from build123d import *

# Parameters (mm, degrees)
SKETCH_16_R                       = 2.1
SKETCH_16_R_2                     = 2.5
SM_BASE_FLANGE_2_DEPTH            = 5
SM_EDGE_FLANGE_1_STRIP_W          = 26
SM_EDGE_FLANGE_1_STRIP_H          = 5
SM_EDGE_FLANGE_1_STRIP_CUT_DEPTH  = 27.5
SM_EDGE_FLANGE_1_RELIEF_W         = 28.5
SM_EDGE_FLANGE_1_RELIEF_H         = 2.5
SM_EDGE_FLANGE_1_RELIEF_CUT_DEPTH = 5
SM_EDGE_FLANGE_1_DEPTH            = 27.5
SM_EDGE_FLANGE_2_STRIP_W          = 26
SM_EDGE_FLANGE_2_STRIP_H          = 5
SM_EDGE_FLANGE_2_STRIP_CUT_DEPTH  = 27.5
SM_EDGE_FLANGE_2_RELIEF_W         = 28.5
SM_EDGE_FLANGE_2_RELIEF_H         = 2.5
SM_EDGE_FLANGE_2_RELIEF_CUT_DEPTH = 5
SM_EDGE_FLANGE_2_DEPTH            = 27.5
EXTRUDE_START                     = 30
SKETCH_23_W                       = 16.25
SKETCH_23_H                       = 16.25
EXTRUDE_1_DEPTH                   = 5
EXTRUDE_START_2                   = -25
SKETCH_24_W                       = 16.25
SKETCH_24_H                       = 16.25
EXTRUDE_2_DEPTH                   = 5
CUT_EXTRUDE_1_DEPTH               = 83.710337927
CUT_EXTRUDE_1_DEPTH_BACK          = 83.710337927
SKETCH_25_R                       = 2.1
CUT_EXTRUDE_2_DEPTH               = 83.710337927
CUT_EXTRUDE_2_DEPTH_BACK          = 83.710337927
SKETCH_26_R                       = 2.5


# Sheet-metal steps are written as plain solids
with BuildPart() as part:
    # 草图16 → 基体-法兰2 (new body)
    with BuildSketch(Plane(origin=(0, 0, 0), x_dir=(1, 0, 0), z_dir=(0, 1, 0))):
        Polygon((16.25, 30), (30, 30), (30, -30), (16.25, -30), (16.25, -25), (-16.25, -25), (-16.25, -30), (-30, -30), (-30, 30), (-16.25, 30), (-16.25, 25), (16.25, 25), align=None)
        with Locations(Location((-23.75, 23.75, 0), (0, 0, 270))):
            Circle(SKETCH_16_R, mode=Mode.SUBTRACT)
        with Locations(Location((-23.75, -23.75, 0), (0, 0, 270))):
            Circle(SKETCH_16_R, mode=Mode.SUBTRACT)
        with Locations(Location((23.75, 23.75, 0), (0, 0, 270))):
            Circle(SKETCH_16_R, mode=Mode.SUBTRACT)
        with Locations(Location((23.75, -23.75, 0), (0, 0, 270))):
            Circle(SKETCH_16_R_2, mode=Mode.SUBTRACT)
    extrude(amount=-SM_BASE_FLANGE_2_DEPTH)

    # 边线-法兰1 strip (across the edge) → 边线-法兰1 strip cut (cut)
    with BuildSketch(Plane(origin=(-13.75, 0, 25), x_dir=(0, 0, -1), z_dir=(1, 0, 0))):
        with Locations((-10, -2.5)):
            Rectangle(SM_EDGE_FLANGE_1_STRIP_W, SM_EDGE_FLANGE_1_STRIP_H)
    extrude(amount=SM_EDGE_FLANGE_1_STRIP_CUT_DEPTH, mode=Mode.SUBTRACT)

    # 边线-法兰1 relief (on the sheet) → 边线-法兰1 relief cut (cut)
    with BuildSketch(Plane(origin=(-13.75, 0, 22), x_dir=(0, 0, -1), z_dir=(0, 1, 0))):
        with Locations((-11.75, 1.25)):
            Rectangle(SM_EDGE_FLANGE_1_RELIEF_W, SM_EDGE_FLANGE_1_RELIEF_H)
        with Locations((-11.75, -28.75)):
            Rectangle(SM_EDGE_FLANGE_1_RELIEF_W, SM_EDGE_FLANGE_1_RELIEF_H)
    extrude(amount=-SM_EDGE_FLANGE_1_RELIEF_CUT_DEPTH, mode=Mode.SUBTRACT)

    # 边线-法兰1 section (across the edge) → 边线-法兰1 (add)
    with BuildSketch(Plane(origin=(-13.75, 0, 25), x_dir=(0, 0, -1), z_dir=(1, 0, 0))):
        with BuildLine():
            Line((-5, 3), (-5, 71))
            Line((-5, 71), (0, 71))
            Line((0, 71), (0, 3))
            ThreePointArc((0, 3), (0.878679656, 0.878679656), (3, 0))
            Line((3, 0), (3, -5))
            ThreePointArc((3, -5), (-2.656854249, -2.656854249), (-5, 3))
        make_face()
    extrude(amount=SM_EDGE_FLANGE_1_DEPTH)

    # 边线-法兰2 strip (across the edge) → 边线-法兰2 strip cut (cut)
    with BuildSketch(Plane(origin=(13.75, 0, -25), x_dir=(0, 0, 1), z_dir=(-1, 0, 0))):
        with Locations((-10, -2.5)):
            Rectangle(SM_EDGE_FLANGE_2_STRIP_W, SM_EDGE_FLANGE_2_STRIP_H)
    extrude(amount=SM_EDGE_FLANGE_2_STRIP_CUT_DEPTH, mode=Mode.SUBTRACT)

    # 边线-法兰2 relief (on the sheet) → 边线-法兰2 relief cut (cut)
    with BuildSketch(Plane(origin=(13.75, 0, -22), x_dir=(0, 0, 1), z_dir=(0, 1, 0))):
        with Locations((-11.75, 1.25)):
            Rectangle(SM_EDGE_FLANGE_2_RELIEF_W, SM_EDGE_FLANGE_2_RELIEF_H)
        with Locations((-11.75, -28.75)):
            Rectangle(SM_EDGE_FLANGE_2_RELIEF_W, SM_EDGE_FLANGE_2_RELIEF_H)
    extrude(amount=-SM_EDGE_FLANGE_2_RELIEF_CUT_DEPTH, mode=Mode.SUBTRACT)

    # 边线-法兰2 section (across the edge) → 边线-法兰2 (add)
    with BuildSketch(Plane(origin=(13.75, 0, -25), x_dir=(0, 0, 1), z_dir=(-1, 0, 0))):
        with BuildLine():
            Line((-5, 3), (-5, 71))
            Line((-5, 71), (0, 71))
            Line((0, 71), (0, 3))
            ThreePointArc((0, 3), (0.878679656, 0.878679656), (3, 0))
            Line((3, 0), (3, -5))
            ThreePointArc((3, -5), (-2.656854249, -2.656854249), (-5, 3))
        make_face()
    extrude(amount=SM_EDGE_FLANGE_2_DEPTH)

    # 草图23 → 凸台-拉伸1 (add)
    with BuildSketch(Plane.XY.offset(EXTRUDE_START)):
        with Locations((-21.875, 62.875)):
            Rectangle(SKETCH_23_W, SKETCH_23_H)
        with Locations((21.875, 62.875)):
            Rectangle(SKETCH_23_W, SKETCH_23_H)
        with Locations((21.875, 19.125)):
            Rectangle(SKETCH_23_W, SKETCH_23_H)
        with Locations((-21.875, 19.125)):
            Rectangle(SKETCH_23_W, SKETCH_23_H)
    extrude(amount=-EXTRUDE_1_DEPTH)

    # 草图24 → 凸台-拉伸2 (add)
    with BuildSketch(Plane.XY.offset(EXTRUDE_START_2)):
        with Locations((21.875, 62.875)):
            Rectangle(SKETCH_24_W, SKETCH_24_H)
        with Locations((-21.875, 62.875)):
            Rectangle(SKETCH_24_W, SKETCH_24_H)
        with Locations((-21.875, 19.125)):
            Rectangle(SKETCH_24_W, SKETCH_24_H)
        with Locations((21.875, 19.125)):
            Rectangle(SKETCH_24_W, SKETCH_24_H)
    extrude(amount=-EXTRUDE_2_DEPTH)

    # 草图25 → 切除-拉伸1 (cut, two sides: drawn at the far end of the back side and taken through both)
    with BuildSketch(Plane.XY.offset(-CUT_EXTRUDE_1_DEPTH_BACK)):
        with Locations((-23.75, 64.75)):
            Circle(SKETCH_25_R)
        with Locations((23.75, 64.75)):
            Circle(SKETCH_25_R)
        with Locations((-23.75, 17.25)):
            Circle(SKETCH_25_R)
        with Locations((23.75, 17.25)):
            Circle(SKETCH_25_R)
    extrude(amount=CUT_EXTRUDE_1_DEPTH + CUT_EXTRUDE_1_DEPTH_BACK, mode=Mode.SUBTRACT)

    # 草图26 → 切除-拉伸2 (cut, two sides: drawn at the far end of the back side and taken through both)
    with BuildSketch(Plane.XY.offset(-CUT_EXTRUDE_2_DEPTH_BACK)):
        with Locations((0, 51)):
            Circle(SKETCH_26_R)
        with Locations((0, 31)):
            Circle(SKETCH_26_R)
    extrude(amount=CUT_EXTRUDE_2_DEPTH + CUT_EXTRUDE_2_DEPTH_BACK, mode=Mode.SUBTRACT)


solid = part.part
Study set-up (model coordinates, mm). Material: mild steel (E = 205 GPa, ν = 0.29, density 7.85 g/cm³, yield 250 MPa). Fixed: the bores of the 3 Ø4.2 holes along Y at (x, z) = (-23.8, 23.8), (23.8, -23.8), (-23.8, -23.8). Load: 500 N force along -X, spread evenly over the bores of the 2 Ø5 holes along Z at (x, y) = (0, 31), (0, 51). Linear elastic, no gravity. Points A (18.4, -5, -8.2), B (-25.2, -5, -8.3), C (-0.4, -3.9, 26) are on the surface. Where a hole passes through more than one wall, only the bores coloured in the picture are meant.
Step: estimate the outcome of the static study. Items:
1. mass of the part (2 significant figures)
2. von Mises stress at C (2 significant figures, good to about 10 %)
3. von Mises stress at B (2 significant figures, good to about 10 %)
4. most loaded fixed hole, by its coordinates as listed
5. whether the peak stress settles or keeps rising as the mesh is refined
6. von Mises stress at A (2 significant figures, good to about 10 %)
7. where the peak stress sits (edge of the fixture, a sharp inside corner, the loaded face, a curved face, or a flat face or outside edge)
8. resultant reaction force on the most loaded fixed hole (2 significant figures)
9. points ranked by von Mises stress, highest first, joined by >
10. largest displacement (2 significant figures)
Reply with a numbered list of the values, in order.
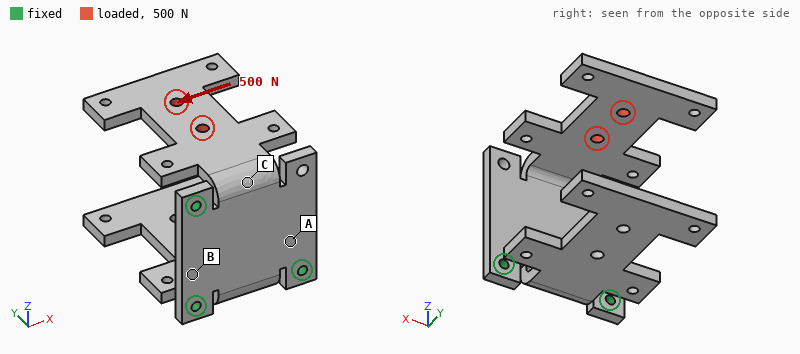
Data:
1. 360 g
2. 81 MPa
3. 19 MPa
4. (23.8, -23.8)
5. keeps rising
6. 55 MPa
7. edge of the fixture
8. 500 N
9. C > A > B
10. 0.46 mm
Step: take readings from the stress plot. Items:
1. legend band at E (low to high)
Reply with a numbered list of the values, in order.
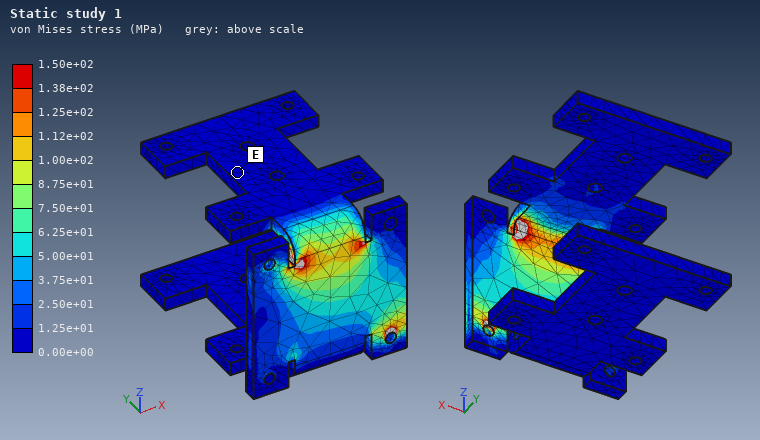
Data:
1. 0.00e+00 to 1.25e+01 MPa
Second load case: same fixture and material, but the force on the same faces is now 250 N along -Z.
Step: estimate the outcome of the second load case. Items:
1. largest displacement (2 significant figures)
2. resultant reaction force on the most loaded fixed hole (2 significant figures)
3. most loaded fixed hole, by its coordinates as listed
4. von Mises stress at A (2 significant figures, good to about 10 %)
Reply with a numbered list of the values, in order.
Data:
1. 0.47 mm
2. 250 N
3. (-23.8, 23.8)
4. 16 MPa
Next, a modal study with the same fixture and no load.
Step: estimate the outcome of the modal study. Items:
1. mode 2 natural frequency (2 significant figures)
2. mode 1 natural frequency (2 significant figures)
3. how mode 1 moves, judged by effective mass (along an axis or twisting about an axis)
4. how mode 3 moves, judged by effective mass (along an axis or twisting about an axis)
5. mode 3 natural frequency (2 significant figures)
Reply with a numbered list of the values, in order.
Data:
1. 440 Hz
2. 420 Hz
3. along Z
4. along X
5. 660 Hz
